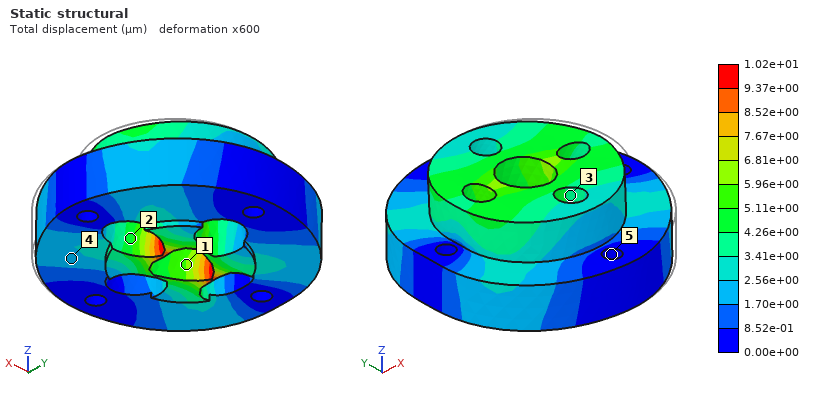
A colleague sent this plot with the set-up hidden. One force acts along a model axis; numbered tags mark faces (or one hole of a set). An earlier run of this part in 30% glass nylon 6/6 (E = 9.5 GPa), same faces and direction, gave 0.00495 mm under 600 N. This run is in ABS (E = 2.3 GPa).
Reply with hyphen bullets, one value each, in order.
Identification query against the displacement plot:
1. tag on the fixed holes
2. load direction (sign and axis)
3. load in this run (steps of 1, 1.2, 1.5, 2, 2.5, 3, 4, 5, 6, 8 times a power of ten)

- 5
- -X
- 300 N
